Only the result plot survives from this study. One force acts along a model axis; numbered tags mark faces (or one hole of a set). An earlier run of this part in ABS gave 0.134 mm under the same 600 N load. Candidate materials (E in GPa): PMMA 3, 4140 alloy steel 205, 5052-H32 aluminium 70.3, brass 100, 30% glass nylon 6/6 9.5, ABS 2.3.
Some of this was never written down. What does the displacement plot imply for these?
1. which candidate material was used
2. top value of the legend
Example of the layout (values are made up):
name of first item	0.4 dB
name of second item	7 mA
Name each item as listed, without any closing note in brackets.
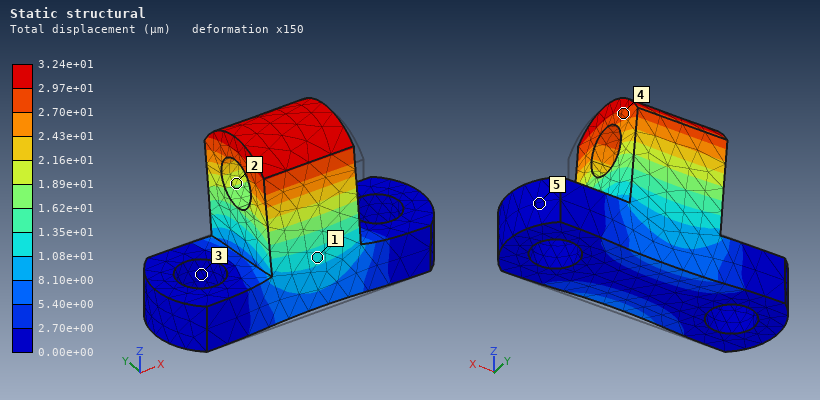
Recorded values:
which candidate material was used	30% glass nylon 6/6
top value of the legend	3.24e+01 µm
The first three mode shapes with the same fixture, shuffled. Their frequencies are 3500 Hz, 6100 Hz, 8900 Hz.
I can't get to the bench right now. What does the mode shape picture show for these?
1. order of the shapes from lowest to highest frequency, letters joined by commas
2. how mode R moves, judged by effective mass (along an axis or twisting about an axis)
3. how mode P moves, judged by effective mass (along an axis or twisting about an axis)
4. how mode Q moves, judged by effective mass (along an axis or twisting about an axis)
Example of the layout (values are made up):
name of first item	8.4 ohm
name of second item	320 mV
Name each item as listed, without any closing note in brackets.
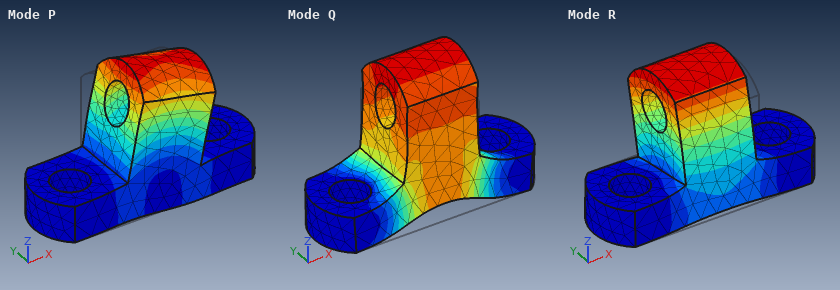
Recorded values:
order of the shapes from lowest to highest frequency, letters joined by commas	R, P, Q
how mode R moves, judged by effective mass	along Y
how mode P moves, judged by effective mass	along X
how mode Q moves, judged by effective mass	along Z
